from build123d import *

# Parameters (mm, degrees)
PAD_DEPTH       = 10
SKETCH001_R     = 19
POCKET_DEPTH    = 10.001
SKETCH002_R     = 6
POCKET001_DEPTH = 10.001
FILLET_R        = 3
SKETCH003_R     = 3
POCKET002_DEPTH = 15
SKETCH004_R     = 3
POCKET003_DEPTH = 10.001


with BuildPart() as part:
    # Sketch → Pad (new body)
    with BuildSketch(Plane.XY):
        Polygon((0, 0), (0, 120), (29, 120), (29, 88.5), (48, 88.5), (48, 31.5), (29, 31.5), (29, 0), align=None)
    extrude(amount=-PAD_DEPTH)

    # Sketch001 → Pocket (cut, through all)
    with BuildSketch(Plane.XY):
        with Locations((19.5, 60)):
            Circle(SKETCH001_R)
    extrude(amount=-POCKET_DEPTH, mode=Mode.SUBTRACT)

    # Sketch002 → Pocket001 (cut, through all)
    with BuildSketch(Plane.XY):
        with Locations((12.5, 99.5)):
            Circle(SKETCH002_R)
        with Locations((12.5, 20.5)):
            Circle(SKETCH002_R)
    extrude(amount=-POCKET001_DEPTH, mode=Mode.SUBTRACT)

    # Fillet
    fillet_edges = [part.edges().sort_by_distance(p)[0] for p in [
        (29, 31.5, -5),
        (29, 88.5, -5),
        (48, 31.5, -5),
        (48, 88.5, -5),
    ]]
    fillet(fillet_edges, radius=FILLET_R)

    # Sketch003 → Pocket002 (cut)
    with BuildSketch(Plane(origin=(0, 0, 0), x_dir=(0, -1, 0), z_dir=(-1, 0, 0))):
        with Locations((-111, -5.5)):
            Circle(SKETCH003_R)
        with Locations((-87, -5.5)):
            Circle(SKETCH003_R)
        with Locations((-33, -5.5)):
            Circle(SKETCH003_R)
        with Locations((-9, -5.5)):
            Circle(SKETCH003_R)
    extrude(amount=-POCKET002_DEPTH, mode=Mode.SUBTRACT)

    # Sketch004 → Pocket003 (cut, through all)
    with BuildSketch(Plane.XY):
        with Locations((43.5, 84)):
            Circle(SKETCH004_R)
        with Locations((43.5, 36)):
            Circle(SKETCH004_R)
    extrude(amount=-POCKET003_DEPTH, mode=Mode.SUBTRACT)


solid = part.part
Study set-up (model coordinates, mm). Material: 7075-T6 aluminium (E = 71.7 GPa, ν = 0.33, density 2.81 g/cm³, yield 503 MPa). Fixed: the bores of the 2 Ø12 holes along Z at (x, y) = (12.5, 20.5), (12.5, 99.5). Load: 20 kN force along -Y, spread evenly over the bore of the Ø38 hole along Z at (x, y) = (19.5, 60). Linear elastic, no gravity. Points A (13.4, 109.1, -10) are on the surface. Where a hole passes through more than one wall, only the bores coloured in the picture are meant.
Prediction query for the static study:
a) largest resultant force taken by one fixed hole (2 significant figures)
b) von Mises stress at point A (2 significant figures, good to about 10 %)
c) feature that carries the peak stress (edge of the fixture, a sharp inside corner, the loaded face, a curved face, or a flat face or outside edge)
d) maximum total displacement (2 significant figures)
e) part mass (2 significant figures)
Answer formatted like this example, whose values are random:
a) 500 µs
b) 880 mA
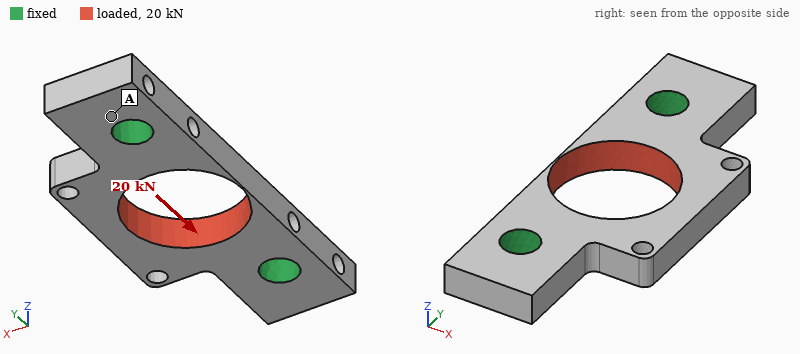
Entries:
a) 10 kN
b) 19 MPa
c) a curved face
d) 45 µm
e) 84 g
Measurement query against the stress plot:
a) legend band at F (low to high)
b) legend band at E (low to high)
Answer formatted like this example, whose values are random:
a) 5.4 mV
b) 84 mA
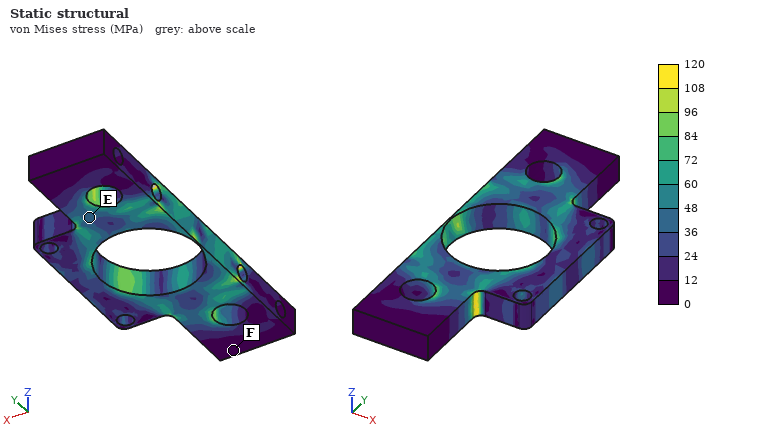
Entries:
a) 0 to 12 MPa
b) 36 to 48 MPa
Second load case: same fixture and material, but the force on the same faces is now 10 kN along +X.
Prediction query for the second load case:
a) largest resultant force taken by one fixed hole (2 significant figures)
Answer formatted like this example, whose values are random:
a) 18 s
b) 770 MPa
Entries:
a) 5.0 kN
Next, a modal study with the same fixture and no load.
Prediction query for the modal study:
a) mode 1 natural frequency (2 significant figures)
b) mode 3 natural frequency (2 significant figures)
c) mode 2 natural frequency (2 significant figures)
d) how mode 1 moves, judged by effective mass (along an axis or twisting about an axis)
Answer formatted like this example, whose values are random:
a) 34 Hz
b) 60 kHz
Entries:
a) 4800 Hz
b) 13 kHz
c) 10 kHz
d) along Z
